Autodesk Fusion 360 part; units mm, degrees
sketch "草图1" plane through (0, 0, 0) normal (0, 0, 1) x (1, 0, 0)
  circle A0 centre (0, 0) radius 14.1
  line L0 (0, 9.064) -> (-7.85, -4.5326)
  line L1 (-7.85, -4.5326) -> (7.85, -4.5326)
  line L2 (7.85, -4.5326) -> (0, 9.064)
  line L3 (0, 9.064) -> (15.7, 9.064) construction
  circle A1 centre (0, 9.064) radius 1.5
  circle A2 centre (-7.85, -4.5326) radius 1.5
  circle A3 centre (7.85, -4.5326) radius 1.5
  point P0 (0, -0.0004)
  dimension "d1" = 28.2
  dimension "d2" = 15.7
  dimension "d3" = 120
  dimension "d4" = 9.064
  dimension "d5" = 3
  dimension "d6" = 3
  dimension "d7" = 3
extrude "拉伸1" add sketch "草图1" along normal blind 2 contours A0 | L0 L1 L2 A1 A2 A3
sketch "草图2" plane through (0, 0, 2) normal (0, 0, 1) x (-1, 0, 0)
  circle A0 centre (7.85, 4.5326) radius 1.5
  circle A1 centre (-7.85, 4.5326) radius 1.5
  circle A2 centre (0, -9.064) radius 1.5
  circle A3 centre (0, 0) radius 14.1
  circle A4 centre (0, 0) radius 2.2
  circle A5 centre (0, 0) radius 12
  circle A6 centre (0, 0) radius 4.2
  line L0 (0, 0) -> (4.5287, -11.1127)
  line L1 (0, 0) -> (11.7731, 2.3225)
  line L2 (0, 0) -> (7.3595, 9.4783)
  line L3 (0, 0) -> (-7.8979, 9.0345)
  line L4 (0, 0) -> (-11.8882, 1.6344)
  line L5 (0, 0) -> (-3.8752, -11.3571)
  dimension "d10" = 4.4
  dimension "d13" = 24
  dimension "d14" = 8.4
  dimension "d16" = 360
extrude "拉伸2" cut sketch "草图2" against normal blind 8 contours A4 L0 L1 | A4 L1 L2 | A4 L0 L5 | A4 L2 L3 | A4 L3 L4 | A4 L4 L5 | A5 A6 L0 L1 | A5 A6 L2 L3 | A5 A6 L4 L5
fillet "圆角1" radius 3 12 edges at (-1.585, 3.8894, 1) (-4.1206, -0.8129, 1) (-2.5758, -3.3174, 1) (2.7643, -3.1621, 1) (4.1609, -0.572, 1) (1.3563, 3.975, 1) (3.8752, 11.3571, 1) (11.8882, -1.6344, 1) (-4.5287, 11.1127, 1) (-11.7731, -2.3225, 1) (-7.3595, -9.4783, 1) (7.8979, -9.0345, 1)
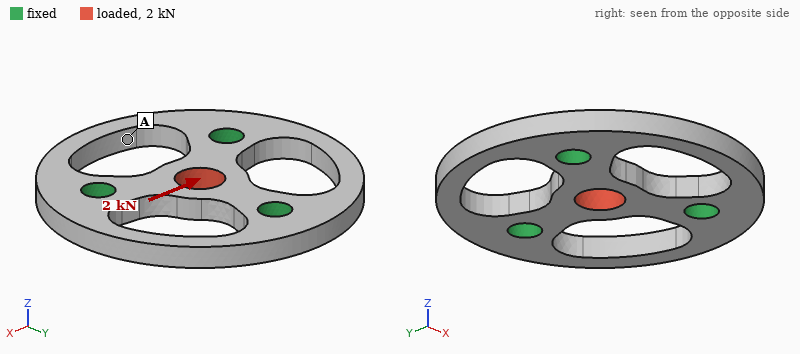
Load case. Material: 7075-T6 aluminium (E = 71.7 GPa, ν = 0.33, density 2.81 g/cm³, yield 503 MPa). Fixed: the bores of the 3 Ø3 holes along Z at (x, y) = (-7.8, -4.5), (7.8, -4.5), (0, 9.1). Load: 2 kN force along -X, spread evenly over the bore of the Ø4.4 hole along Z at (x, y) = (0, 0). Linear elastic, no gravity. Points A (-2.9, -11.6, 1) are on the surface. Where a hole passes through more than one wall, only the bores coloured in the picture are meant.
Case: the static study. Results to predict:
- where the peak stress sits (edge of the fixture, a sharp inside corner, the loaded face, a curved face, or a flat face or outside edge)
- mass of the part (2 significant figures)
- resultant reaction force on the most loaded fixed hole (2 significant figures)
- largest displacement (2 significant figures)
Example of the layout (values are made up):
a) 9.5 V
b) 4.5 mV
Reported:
a) the loaded face
b) 2.0 g
c) 840 N
d) 26 µm
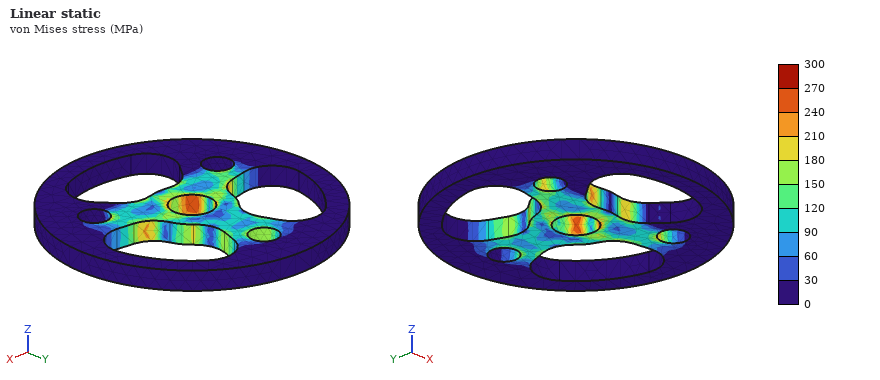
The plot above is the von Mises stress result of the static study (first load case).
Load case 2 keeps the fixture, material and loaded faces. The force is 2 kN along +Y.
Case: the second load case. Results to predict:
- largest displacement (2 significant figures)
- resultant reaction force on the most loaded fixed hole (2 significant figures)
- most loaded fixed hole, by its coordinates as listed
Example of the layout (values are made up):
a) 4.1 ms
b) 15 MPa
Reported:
a) 28 µm
b) 950 N
c) (0, 9.1)
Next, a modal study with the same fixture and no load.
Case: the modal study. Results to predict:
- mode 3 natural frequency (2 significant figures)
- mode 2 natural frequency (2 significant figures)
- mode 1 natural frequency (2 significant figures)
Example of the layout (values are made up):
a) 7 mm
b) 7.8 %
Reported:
a) 19 kHz
b) 18 kHz
c) 18 kHz
